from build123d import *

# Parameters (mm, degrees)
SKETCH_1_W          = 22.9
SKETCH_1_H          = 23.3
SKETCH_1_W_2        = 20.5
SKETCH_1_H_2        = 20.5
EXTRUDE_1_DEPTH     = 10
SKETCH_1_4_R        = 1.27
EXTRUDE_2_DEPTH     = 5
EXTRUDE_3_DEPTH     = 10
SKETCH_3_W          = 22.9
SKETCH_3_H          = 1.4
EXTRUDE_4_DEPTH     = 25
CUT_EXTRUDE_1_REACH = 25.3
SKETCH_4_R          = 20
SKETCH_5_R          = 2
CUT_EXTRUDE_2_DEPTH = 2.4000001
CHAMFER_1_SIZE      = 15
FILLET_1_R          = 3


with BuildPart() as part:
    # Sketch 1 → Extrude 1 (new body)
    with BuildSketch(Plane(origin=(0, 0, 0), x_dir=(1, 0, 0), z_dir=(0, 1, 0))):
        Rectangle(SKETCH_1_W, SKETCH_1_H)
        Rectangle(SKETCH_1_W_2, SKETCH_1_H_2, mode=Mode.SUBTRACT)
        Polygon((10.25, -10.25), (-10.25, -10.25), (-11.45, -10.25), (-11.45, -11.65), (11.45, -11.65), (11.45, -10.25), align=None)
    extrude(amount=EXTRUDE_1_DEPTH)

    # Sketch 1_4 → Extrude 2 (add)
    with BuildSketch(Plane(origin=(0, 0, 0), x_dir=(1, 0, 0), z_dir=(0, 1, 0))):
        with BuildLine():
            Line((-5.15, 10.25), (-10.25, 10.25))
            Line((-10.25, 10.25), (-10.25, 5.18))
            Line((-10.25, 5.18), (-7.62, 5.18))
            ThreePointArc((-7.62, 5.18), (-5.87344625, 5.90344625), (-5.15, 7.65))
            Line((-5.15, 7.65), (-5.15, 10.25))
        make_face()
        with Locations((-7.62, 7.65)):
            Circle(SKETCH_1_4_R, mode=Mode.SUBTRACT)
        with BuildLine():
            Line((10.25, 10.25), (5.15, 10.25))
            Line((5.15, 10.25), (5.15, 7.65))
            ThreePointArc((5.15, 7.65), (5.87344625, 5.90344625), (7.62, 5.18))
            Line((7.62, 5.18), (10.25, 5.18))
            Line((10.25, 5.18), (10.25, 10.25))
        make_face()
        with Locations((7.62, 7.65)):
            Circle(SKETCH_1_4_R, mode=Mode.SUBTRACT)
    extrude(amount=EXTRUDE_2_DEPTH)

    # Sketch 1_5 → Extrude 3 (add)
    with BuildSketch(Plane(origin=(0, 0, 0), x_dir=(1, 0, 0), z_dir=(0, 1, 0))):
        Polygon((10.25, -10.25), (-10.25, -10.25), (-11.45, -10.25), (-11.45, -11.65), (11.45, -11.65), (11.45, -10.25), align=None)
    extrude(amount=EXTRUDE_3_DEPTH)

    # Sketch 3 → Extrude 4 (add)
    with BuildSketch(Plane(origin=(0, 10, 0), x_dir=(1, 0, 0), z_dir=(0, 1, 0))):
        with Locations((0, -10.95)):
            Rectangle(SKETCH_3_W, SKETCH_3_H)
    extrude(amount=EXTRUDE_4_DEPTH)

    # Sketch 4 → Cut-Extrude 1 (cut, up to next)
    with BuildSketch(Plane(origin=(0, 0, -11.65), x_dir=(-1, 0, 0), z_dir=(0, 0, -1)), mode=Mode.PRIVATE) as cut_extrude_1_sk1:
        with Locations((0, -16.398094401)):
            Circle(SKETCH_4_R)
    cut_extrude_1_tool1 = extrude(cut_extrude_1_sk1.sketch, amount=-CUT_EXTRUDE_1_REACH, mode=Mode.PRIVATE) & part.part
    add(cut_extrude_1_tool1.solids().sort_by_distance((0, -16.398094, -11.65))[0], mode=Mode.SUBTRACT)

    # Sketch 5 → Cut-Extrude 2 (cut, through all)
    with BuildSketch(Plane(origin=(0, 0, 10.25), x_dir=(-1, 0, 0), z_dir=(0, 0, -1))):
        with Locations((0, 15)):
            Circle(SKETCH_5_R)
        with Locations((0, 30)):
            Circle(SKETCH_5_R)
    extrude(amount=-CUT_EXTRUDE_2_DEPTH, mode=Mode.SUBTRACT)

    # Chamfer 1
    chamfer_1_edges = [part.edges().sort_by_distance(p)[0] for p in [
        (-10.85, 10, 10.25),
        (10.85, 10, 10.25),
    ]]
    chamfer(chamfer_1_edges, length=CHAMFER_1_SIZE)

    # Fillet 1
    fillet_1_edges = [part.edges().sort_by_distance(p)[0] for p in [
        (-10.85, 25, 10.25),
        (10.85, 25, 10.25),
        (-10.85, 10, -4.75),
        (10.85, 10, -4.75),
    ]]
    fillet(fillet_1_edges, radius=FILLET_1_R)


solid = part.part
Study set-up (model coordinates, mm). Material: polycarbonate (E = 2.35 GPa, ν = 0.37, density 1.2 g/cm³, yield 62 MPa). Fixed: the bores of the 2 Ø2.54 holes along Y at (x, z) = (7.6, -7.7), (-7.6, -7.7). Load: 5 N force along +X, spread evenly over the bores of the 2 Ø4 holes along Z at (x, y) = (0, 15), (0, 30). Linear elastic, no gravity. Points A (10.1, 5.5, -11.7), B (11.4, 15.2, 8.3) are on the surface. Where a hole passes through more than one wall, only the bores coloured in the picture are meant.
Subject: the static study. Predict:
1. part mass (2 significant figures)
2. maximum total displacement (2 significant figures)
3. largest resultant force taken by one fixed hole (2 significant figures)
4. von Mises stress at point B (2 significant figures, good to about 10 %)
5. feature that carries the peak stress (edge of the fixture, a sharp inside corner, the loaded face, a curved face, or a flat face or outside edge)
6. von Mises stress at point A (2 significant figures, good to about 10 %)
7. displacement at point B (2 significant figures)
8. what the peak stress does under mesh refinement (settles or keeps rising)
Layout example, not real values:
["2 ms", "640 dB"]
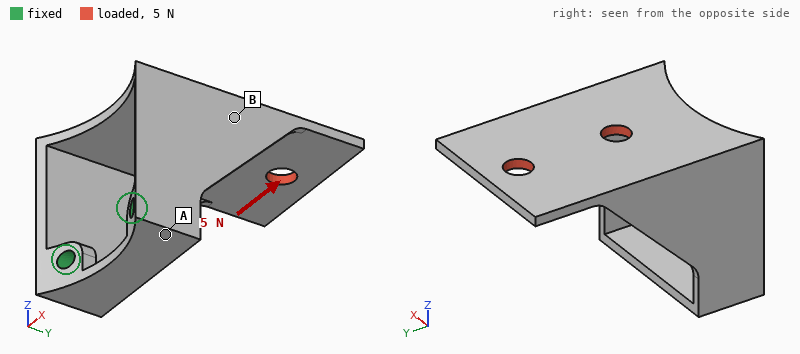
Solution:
["2.5 g", "0.48 mm", "4.7 N", "3.3 MPa", "edge of the fixture", "0.91 MPa", "0.34 mm", "keeps rising"]
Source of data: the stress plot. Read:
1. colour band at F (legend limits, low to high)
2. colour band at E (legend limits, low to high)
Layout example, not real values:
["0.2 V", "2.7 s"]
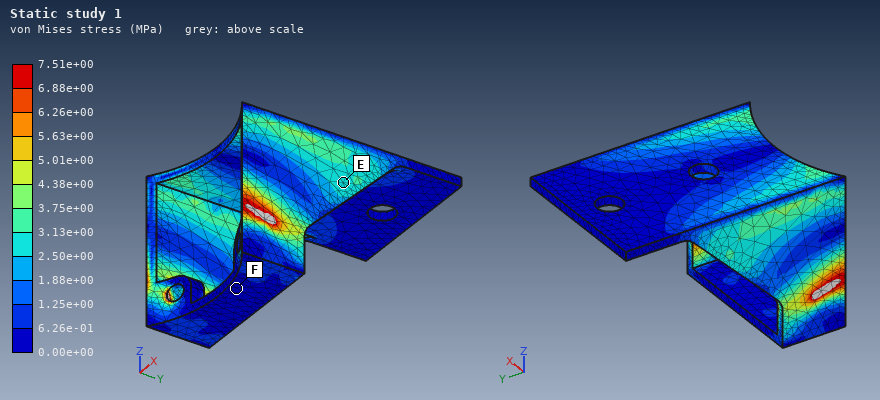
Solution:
["0.00e+00 to 6.26e-01 MPa", "2.50e+00 to 3.13e+00 MPa"]
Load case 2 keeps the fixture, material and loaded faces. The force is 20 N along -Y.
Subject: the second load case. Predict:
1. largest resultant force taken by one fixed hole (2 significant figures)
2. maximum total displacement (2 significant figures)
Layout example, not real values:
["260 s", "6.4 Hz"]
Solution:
["10 N", "0.56 mm"]
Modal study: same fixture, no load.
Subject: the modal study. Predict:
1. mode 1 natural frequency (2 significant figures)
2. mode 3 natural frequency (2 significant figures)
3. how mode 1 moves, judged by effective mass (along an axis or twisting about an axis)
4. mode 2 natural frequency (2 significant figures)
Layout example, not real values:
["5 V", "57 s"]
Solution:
["480 Hz", "1100 Hz", "along X", "750 Hz"]
